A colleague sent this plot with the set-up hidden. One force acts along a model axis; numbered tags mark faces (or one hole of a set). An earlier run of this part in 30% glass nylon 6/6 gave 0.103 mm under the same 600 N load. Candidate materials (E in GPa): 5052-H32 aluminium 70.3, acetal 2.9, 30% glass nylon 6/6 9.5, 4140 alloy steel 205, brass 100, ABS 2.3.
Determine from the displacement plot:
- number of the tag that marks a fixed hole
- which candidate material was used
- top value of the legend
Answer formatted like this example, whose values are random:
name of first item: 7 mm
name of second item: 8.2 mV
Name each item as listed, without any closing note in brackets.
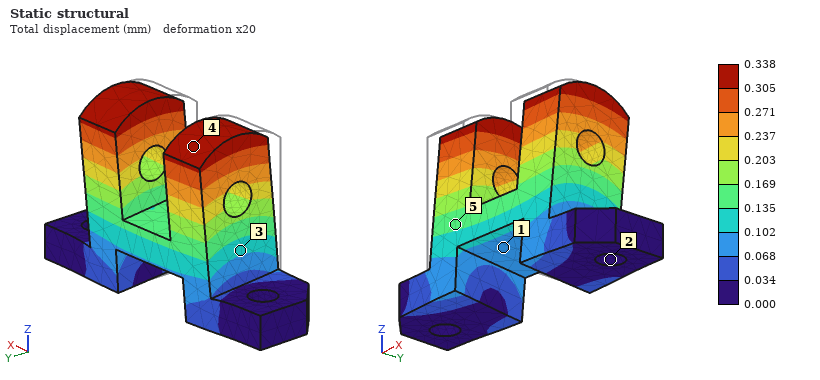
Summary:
number of the tag that marks a fixed hole: 2
which candidate material was used: acetal
top value of the legend: 0.338 mm
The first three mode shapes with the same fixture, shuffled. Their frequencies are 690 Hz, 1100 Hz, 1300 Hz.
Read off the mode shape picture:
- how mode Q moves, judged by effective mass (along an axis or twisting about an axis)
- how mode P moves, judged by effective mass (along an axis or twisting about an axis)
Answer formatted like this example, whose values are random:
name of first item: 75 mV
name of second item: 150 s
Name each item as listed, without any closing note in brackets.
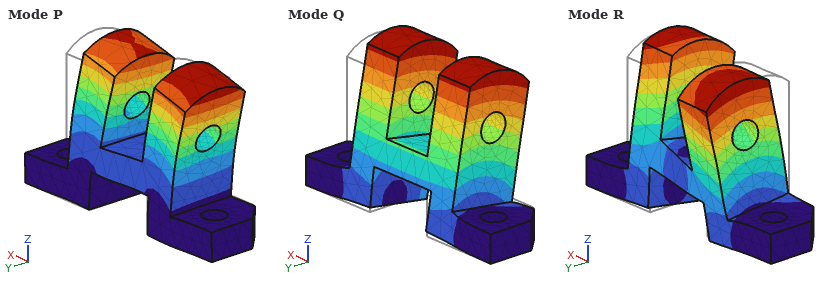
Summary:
how mode Q moves, judged by effective mass: along Y
how mode P moves, judged by effective mass: along X
